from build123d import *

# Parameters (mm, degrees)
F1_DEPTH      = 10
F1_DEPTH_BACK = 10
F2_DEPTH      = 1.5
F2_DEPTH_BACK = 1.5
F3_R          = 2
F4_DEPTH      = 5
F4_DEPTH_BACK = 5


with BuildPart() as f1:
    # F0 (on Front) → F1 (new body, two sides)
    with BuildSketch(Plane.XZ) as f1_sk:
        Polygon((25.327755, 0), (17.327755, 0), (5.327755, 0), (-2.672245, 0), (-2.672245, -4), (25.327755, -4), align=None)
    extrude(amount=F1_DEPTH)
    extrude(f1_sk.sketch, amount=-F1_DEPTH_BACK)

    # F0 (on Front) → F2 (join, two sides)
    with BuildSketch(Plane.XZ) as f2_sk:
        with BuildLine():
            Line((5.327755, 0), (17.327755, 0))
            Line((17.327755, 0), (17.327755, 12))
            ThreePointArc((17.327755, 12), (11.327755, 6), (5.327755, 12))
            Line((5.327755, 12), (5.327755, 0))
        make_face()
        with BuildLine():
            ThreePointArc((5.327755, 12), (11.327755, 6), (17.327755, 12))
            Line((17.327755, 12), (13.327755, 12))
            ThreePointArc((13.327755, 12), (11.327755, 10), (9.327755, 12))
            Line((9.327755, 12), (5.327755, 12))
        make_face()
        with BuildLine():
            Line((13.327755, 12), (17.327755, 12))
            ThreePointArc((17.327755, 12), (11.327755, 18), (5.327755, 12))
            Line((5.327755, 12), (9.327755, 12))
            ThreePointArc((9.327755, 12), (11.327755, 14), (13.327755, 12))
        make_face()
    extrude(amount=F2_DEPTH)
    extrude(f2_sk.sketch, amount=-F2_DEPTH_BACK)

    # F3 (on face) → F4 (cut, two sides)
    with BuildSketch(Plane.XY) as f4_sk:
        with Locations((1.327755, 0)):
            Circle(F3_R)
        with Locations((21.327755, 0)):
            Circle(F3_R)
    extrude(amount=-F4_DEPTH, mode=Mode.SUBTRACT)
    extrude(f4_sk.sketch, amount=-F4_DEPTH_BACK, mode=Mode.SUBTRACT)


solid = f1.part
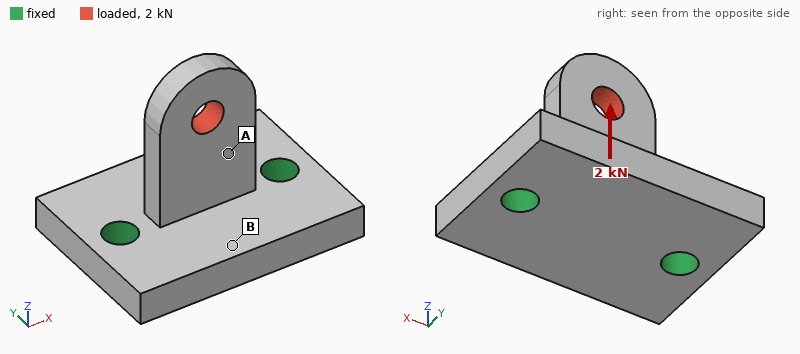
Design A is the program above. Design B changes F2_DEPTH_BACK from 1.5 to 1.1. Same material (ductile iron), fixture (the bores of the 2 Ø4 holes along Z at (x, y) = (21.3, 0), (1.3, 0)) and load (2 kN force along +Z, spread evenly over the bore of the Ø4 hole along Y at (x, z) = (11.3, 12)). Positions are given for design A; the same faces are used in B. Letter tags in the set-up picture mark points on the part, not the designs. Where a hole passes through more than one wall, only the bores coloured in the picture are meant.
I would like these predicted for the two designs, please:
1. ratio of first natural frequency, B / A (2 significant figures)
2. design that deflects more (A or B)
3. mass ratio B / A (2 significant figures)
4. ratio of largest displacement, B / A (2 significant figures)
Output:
0.90
B
0.97
1.1
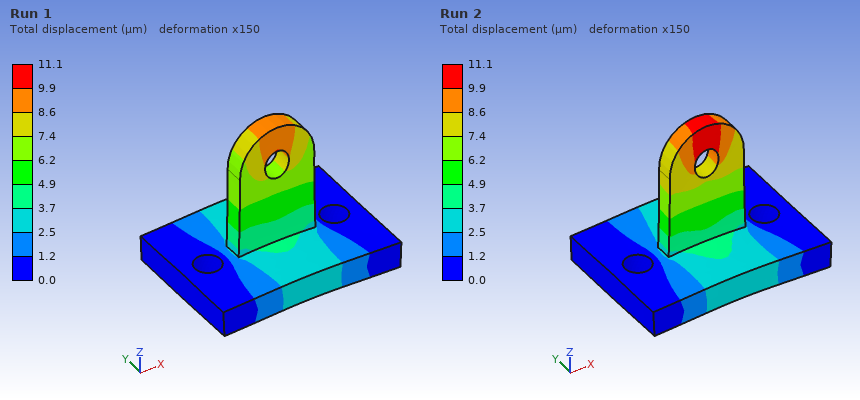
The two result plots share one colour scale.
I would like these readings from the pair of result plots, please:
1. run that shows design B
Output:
Run 2
